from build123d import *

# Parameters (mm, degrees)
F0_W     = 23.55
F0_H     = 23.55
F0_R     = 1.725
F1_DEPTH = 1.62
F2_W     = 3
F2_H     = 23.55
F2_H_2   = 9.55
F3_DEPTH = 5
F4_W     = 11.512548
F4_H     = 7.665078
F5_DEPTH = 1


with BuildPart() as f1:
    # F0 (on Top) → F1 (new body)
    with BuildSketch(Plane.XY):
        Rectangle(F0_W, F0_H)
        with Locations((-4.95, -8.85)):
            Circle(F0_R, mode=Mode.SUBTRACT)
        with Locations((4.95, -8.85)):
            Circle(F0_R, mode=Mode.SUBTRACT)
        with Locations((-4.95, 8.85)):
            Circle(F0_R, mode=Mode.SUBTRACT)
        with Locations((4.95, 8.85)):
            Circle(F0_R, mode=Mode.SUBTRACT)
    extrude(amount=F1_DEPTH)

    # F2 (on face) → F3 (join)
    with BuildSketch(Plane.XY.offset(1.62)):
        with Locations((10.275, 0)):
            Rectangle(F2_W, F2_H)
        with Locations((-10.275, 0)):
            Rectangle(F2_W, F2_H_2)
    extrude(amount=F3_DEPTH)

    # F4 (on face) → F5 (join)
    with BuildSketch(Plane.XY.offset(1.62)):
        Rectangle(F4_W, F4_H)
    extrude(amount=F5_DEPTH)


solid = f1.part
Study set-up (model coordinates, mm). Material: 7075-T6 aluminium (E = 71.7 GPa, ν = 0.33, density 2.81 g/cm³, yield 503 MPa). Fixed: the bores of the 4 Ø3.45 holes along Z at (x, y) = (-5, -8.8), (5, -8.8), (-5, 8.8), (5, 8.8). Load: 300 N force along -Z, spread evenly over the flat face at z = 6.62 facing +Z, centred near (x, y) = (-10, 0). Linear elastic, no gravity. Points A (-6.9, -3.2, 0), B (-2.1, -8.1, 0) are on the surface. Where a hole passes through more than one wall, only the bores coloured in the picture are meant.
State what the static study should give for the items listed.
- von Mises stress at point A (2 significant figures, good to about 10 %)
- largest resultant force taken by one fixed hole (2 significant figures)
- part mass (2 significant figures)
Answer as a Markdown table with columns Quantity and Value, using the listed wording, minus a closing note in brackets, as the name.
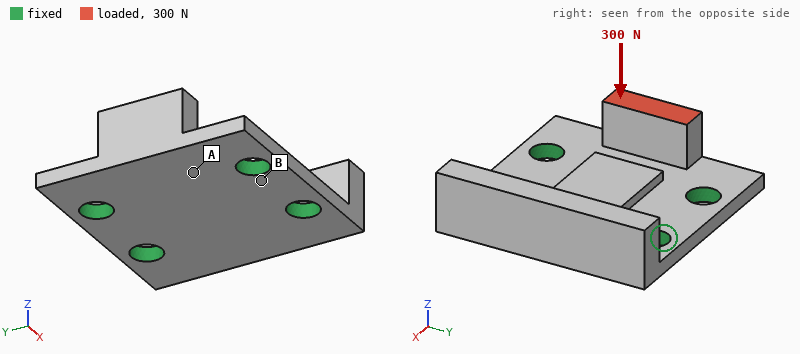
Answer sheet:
| Quantity | Value |
|---|---|
| von Mises stress at point A | 71 MPa |
| largest resultant force taken by one fixed hole | 180 N |
| part mass | 4.0 g |
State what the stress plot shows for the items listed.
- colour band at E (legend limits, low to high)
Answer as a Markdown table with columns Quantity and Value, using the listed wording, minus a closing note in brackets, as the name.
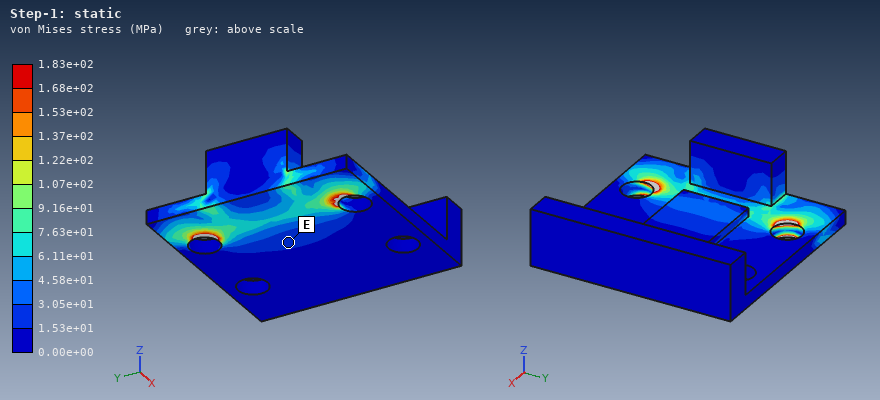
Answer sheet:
| Quantity | Value |
|---|---|
| colour band at E | 1.53e+01 to 3.05e+01 MPa |
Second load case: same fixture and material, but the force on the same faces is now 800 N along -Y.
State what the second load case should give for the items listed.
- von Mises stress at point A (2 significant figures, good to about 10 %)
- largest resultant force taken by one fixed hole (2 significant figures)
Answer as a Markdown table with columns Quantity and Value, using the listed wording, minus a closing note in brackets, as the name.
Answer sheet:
| Quantity | Value |
|---|---|
| von Mises stress at point A | 89 MPa |
| largest resultant force taken by one fixed hole | 550 N |
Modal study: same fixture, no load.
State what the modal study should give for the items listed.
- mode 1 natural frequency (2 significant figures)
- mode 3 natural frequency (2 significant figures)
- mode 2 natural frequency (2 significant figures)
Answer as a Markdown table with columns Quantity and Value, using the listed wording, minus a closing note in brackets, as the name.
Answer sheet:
| Quantity | Value |
|---|---|
| mode 1 natural frequency | 13 kHz |
| mode 3 natural frequency | 26 kHz |
| mode 2 natural frequency | 16 kHz |
